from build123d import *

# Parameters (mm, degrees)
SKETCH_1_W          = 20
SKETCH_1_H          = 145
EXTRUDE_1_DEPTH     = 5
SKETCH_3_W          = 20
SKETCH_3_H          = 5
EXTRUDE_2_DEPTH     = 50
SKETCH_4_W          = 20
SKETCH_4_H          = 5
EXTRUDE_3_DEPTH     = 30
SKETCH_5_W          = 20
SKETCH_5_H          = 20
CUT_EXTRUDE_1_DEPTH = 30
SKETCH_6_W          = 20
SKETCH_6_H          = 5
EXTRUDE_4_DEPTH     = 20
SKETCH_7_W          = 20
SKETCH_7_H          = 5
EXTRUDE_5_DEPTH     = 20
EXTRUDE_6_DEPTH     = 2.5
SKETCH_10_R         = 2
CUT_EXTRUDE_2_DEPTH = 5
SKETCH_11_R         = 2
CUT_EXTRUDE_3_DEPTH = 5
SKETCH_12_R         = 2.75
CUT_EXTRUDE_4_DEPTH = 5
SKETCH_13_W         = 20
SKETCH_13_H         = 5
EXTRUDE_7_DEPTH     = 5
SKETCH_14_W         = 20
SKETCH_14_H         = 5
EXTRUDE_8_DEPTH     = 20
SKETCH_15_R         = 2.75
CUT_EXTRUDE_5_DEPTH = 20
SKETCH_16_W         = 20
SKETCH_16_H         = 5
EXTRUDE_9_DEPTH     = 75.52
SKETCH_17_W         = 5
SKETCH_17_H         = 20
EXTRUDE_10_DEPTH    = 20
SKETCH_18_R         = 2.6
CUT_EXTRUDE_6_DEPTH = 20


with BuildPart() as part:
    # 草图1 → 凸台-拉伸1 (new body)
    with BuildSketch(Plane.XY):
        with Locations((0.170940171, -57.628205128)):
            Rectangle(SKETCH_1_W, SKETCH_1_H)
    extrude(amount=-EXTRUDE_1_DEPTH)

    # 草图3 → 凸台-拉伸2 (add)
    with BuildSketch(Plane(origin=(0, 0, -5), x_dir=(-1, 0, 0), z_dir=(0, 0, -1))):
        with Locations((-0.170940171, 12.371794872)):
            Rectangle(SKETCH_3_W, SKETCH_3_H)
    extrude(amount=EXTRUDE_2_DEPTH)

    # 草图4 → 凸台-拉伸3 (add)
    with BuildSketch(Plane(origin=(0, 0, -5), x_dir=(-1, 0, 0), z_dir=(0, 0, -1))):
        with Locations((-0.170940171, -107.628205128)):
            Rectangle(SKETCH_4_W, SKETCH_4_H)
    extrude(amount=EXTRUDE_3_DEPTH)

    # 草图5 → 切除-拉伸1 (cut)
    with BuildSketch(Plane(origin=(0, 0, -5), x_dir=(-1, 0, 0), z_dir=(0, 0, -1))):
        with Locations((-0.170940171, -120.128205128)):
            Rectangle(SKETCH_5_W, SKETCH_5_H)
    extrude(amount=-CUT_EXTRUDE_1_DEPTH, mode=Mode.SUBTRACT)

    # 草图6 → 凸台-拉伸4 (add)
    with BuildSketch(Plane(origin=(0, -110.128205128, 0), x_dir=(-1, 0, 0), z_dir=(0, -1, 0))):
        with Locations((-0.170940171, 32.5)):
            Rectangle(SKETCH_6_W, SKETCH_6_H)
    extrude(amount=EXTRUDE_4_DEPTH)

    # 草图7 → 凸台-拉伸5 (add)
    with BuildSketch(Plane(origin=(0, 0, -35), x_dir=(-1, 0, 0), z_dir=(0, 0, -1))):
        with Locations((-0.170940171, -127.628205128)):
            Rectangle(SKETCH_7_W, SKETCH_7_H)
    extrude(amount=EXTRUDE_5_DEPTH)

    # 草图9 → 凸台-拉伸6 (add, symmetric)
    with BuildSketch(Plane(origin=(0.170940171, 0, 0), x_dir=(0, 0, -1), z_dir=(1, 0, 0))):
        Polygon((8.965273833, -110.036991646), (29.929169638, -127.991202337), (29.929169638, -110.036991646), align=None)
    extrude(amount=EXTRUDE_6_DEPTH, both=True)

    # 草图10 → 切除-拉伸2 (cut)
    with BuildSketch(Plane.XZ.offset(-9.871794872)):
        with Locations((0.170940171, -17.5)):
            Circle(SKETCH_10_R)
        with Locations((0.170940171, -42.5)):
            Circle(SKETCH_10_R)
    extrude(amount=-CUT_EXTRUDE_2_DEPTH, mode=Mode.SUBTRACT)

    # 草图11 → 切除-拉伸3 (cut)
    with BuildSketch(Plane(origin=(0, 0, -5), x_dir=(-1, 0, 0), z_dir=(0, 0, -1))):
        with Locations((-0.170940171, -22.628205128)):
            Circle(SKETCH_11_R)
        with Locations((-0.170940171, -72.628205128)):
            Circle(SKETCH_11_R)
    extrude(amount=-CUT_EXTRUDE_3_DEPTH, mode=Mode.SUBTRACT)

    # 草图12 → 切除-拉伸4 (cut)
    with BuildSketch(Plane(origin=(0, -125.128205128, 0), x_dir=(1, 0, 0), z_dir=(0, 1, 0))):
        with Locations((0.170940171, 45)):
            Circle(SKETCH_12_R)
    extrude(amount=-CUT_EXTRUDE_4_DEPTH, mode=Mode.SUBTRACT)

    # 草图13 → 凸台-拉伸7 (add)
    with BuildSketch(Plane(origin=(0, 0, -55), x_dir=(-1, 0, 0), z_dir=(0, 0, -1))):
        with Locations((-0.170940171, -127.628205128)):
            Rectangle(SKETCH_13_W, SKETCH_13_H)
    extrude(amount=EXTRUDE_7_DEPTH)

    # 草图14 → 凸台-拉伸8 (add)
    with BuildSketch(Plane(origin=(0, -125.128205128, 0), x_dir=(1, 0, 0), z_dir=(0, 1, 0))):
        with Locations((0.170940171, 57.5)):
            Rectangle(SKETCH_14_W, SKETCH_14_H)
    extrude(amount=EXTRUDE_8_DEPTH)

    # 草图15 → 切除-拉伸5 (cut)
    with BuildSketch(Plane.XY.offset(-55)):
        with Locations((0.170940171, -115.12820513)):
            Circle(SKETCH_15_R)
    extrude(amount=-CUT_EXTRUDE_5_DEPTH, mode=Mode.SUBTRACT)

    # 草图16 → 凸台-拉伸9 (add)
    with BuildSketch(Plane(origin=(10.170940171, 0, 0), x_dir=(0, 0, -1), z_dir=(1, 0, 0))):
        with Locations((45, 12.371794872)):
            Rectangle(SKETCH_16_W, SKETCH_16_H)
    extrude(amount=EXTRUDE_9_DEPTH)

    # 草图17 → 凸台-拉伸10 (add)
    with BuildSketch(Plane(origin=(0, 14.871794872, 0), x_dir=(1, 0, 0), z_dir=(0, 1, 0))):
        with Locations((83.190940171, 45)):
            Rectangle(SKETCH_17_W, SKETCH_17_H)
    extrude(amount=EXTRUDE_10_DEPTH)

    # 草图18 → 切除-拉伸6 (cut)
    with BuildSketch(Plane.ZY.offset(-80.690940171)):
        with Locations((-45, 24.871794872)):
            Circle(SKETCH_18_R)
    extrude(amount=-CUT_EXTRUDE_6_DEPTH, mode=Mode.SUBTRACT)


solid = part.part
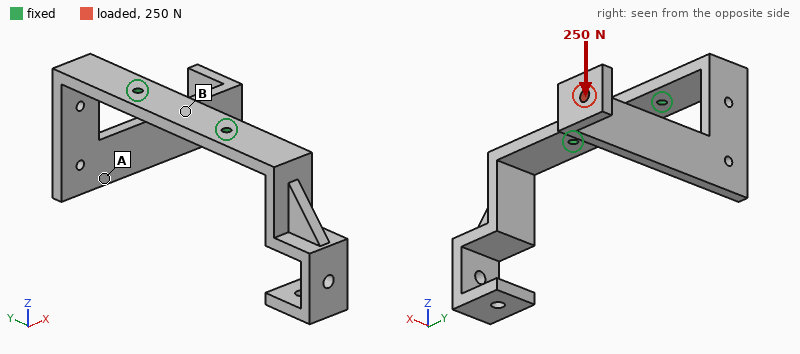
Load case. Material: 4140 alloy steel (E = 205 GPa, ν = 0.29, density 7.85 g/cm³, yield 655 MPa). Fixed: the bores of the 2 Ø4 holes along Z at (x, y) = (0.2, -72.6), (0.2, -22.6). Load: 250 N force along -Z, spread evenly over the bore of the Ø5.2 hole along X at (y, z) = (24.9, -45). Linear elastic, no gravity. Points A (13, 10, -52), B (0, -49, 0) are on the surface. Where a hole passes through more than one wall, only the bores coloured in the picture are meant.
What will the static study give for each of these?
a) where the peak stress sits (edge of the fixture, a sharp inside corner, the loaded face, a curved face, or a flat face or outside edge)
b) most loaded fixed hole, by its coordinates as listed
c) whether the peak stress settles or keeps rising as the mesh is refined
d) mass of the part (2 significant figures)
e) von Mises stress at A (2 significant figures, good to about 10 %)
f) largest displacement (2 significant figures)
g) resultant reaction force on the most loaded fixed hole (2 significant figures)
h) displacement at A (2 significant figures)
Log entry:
edge of the fixture
(0.2, -22.6)
keeps rising
290 g
46 MPa
1.8 mm
280 N
0.79 mm
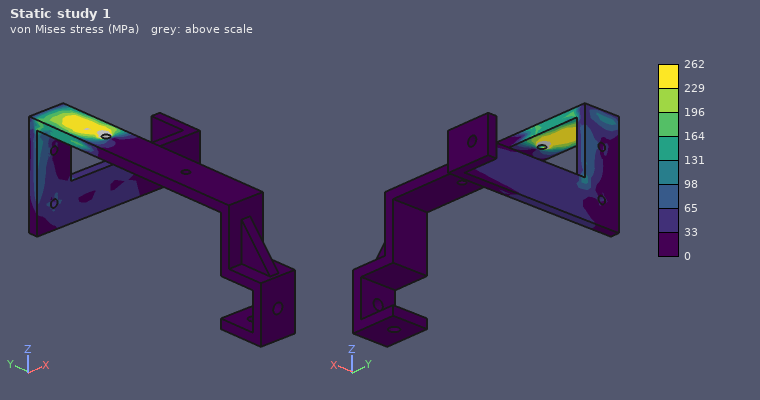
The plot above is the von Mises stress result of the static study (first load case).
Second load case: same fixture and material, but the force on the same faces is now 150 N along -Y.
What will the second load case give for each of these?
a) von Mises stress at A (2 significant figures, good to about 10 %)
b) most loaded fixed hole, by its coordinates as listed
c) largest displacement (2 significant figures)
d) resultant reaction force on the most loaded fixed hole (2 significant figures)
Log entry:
110 MPa
(0.2, -22.6)
1.8 mm
230 N
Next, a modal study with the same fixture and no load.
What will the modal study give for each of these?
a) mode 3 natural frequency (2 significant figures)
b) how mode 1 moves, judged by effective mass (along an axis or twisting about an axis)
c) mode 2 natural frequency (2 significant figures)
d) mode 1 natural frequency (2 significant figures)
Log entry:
380 Hz
along Y
300 Hz
230 Hz
